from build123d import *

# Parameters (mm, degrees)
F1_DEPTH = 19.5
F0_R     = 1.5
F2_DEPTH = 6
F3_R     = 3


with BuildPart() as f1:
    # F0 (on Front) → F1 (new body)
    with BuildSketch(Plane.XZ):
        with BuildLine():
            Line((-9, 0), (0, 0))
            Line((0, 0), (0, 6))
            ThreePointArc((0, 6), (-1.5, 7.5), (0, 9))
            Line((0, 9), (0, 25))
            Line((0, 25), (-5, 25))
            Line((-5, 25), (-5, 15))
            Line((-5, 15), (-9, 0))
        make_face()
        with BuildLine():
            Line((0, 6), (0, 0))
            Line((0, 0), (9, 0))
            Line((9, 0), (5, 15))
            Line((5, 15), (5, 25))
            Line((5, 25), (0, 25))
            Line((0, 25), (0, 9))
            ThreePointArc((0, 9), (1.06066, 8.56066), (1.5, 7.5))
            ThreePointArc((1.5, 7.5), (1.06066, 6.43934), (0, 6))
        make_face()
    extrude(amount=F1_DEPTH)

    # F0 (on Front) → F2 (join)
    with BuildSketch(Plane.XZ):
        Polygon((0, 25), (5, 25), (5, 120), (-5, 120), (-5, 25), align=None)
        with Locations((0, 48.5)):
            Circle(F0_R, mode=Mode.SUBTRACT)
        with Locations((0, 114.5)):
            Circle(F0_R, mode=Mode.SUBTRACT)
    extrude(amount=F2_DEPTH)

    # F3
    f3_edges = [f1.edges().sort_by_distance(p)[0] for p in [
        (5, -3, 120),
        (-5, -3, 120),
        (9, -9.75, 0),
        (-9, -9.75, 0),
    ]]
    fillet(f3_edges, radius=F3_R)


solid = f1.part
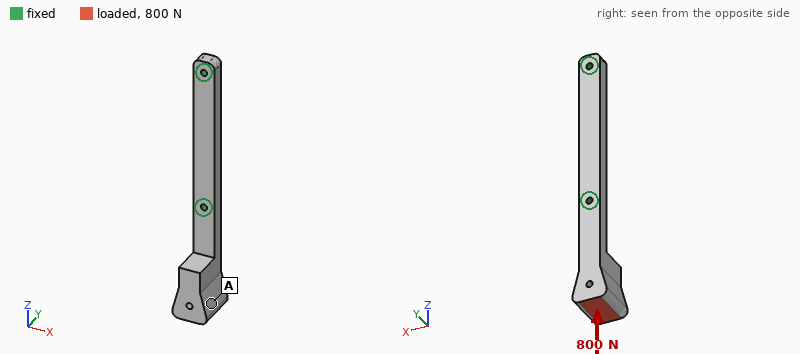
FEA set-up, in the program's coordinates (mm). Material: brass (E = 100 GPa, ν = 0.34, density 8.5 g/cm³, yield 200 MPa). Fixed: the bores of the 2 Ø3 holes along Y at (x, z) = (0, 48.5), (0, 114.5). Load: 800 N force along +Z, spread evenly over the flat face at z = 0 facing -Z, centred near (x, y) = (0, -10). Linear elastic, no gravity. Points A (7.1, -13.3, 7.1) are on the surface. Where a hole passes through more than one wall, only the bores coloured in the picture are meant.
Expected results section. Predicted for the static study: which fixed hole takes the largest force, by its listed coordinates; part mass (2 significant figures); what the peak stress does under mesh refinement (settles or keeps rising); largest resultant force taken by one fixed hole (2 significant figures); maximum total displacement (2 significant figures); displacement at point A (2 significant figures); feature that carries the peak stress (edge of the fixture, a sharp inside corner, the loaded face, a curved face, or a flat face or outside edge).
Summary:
(0, 48.5)
97 g
keeps rising
780 N
0.31 mm
0.24 mm
edge of the fixture
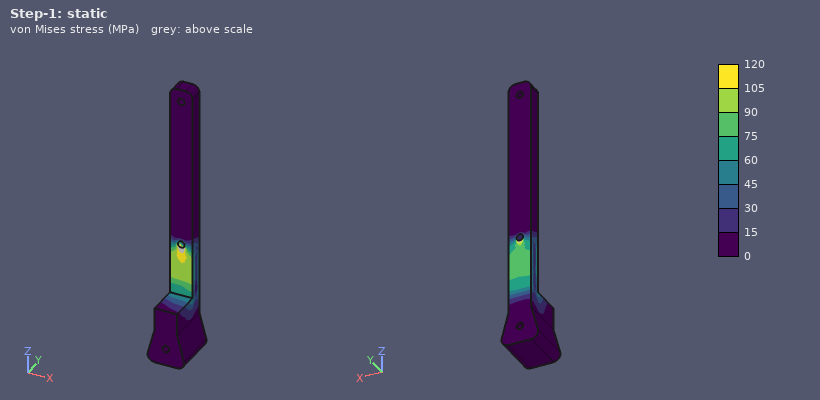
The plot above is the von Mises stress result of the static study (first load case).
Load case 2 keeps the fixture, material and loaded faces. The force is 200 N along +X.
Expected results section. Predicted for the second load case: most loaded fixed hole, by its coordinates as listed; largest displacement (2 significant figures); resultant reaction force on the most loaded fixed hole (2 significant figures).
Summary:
(0, 48.5)
0.22 mm
250 N
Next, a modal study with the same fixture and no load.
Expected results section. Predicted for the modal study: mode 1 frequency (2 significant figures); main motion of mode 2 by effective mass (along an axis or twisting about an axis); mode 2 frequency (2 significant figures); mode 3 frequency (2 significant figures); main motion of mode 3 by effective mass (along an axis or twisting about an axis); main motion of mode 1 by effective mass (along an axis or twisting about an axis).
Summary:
680 Hz
along X
930 Hz
2800 Hz
twisting about Z
along Y
